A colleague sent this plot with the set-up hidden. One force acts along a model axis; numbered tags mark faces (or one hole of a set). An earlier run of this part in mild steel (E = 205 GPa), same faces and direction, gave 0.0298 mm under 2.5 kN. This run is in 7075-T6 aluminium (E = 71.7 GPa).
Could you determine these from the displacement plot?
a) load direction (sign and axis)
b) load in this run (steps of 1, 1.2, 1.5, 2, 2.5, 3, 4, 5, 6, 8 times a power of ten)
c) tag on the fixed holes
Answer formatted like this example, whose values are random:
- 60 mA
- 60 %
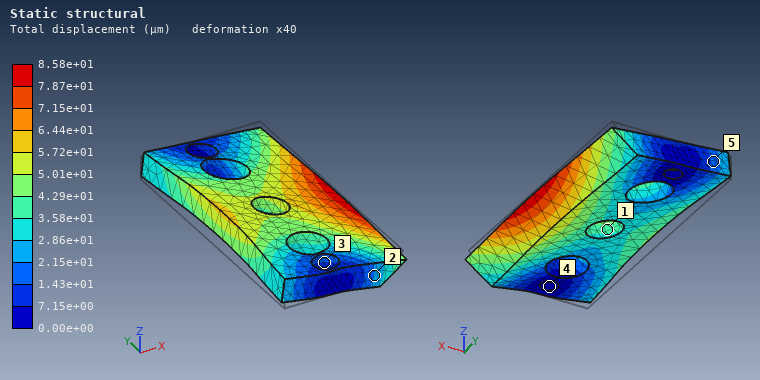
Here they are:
- +X
- 2.5 kN
- 4
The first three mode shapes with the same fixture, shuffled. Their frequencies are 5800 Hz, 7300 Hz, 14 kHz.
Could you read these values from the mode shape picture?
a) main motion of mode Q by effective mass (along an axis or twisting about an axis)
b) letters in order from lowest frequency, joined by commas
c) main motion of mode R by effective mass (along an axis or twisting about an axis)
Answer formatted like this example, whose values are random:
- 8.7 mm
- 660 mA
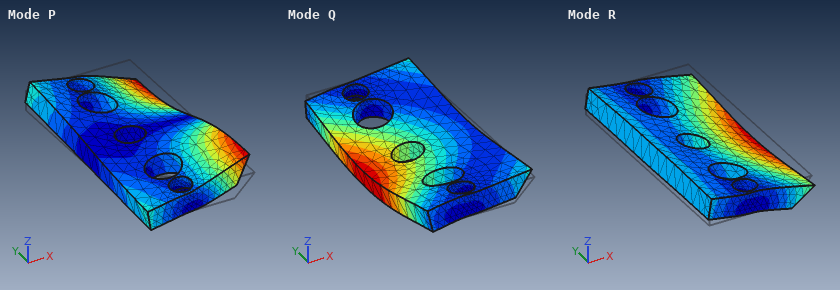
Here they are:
- along Z
- R, Q, P
- along Z
